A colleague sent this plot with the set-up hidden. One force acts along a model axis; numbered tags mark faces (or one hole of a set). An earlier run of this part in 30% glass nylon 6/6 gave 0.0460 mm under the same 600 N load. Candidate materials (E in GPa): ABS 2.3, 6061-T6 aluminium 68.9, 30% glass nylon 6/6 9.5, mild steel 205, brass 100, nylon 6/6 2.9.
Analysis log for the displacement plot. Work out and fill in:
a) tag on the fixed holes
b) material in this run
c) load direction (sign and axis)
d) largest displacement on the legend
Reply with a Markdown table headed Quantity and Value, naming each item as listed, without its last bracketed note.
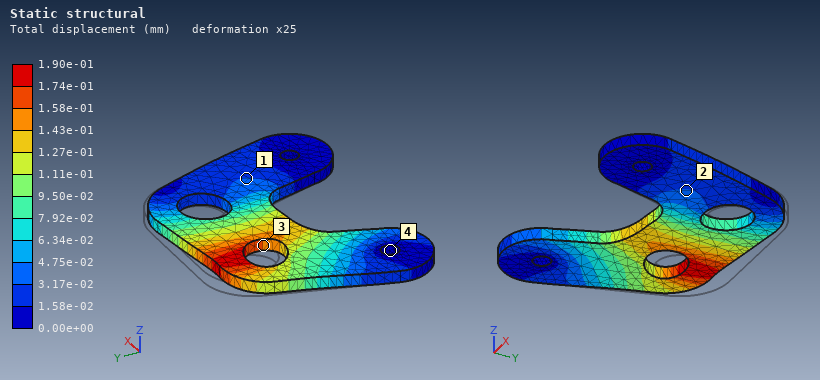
| Quantity | Value |
|---|---|
| tag on the fixed holes | 4 |
| material in this run | ABS |
| load direction | -Y |
| largest displacement on the legend | 1.90e-01 mm |
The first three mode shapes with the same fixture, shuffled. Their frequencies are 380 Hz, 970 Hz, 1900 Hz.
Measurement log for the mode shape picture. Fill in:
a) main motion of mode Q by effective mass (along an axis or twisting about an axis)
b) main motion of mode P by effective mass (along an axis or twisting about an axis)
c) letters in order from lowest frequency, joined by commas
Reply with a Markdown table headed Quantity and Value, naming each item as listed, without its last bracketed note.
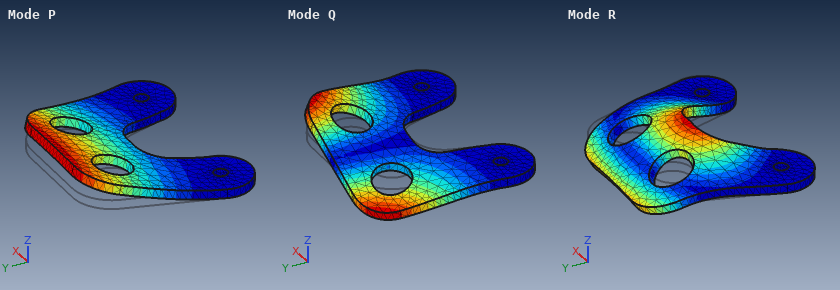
| Quantity | Value |
|---|---|
| main motion of mode Q by effective mass | twisting about Y |
| main motion of mode P by effective mass | along Z |
| letters in order from lowest frequency, joined by commas | P, Q, R |
